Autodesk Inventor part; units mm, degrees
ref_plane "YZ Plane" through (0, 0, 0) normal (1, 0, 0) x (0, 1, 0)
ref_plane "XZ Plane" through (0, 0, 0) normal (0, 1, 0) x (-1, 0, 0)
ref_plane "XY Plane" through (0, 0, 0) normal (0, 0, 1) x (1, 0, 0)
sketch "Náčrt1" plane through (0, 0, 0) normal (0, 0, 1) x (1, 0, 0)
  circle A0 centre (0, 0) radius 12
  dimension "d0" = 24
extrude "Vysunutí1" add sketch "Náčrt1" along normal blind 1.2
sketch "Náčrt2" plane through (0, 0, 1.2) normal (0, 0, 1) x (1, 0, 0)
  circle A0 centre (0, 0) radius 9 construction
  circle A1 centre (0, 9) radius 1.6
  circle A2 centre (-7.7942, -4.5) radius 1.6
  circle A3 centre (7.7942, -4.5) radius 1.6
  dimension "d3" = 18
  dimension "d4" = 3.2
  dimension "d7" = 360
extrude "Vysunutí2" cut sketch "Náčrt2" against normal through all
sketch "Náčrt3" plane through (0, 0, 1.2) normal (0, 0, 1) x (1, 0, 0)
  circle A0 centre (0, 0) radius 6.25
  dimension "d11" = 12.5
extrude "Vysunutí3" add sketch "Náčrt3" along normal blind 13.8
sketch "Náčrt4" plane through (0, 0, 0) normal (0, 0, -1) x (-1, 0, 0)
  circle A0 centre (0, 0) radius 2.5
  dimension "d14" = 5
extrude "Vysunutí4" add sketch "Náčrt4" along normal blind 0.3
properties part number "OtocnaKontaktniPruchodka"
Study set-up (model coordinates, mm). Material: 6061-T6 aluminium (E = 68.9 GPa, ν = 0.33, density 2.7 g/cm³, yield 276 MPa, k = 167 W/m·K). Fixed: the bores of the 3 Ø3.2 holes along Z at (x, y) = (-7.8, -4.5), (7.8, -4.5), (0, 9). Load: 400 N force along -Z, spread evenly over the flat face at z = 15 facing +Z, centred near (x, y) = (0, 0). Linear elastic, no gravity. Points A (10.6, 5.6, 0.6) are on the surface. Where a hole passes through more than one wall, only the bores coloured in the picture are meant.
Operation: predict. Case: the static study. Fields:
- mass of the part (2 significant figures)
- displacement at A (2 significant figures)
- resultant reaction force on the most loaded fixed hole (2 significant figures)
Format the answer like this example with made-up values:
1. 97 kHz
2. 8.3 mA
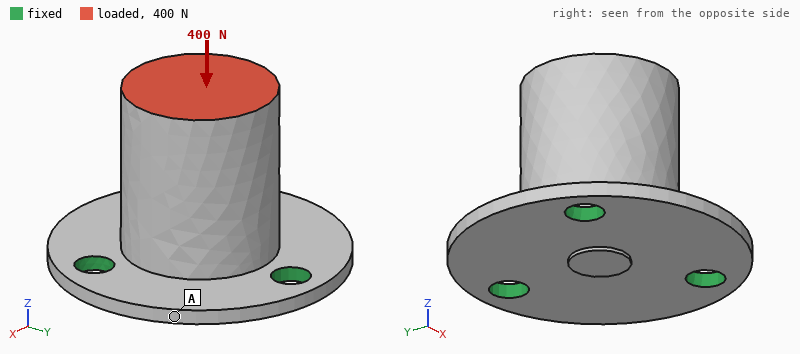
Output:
1. 6.0 g
2. 3.3 µm
3. 150 N
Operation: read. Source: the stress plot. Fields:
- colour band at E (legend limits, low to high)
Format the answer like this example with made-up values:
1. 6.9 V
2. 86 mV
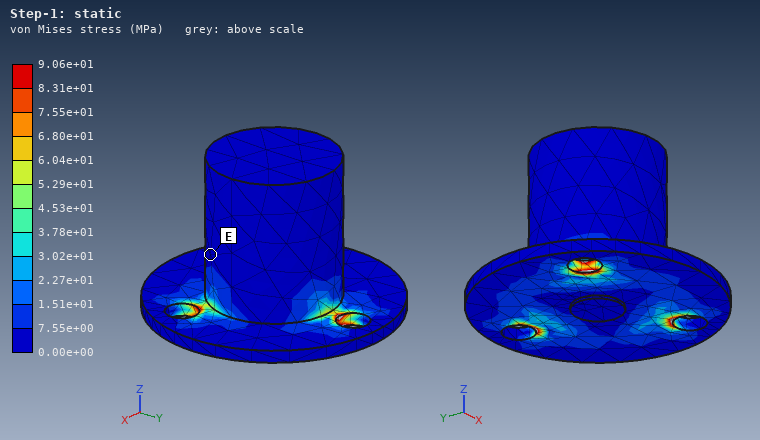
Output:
1. 0.00e+00 to 7.55e+00 MPa
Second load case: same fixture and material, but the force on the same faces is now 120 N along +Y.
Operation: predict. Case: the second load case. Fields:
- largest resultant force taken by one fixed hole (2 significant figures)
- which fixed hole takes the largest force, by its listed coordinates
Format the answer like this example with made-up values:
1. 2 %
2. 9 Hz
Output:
1. 170 N
2. (0, 9)
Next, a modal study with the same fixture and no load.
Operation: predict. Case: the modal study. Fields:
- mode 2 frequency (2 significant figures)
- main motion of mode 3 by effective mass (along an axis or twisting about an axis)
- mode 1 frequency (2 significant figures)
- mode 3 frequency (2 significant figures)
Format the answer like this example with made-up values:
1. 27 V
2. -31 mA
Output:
1. 12 kHz
2. along Z
3. 12 kHz
4. 21 kHz
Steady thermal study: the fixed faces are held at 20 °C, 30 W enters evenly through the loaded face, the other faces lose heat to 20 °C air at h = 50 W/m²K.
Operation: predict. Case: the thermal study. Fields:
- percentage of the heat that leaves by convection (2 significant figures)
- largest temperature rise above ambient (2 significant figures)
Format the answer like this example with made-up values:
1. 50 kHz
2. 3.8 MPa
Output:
1. 3.6 %
2. 36 K
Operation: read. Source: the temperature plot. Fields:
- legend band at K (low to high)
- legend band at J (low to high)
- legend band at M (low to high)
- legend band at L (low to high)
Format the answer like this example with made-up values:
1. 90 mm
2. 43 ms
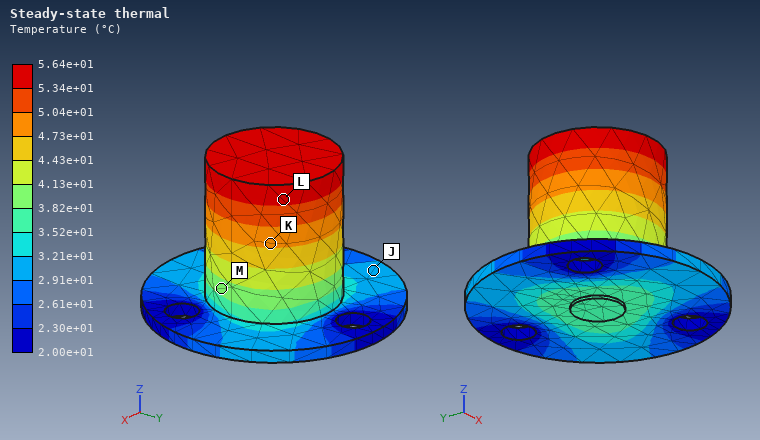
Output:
1. 4.73e+01 to 5.04e+01 °C
2. 2.91e+01 to 3.21e+01 °C
3. 3.82e+01 to 4.13e+01 °C
4. 5.34e+01 to 5.64e+01 °C
